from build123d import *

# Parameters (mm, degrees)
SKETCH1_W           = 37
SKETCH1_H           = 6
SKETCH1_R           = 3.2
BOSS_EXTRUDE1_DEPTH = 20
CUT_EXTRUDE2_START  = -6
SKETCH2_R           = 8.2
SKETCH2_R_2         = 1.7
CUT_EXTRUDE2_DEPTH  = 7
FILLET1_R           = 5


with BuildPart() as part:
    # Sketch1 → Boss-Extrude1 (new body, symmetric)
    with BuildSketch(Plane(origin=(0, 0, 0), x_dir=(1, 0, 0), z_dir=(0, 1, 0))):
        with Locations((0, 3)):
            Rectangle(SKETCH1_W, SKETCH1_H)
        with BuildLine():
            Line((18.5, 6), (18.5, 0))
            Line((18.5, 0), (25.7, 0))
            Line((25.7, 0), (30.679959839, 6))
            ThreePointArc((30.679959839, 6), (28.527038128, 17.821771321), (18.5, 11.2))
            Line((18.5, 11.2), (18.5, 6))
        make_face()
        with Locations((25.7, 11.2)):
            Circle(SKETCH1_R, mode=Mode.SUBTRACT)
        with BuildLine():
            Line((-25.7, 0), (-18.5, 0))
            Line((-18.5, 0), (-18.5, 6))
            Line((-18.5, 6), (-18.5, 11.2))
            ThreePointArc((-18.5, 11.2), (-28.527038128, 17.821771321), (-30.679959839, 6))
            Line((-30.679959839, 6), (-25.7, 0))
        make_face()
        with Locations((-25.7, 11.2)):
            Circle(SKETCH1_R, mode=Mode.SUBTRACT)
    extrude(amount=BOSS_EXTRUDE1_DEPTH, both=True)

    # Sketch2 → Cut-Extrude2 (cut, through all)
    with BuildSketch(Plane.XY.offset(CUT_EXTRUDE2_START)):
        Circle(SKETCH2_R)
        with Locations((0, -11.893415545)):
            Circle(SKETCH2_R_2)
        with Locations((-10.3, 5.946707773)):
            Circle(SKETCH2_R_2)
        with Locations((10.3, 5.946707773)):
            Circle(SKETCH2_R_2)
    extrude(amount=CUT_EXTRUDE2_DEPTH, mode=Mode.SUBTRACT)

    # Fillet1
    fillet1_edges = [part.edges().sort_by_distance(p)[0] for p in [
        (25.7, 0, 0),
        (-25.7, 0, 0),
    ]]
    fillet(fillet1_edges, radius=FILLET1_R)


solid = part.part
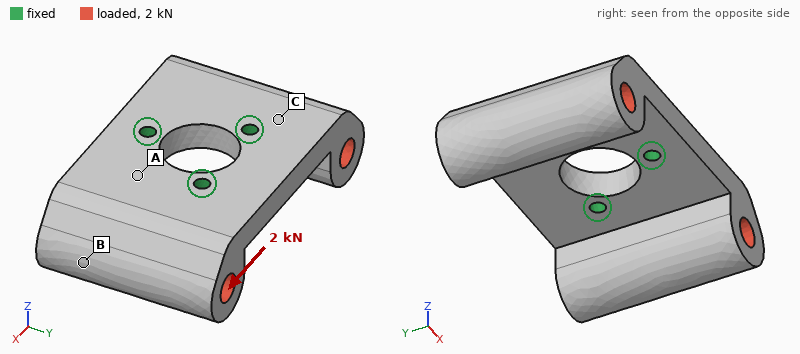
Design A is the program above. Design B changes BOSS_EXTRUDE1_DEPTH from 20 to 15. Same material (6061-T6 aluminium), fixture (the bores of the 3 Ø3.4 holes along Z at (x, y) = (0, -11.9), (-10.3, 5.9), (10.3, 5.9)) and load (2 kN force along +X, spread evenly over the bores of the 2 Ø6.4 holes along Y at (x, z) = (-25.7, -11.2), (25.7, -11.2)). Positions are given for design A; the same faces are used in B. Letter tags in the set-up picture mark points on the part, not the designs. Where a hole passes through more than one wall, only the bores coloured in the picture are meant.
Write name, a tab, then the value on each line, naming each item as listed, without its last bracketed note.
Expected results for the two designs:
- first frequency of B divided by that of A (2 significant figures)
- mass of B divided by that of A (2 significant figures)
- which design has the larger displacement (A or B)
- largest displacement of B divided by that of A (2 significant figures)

first frequency of B divided by that of A	1.0
mass of B divided by that of A	0.73
which design has the larger displacement	B
largest displacement of B divided by that of A	1.3
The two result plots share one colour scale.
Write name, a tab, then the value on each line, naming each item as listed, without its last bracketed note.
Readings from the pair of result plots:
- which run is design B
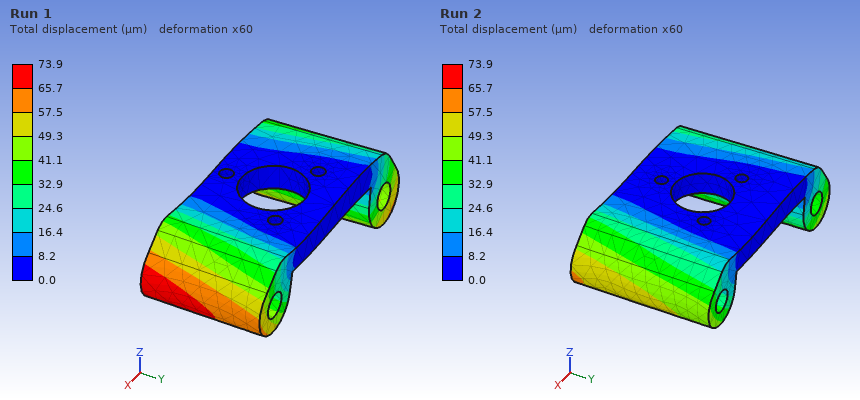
which run is design B	Run 1
